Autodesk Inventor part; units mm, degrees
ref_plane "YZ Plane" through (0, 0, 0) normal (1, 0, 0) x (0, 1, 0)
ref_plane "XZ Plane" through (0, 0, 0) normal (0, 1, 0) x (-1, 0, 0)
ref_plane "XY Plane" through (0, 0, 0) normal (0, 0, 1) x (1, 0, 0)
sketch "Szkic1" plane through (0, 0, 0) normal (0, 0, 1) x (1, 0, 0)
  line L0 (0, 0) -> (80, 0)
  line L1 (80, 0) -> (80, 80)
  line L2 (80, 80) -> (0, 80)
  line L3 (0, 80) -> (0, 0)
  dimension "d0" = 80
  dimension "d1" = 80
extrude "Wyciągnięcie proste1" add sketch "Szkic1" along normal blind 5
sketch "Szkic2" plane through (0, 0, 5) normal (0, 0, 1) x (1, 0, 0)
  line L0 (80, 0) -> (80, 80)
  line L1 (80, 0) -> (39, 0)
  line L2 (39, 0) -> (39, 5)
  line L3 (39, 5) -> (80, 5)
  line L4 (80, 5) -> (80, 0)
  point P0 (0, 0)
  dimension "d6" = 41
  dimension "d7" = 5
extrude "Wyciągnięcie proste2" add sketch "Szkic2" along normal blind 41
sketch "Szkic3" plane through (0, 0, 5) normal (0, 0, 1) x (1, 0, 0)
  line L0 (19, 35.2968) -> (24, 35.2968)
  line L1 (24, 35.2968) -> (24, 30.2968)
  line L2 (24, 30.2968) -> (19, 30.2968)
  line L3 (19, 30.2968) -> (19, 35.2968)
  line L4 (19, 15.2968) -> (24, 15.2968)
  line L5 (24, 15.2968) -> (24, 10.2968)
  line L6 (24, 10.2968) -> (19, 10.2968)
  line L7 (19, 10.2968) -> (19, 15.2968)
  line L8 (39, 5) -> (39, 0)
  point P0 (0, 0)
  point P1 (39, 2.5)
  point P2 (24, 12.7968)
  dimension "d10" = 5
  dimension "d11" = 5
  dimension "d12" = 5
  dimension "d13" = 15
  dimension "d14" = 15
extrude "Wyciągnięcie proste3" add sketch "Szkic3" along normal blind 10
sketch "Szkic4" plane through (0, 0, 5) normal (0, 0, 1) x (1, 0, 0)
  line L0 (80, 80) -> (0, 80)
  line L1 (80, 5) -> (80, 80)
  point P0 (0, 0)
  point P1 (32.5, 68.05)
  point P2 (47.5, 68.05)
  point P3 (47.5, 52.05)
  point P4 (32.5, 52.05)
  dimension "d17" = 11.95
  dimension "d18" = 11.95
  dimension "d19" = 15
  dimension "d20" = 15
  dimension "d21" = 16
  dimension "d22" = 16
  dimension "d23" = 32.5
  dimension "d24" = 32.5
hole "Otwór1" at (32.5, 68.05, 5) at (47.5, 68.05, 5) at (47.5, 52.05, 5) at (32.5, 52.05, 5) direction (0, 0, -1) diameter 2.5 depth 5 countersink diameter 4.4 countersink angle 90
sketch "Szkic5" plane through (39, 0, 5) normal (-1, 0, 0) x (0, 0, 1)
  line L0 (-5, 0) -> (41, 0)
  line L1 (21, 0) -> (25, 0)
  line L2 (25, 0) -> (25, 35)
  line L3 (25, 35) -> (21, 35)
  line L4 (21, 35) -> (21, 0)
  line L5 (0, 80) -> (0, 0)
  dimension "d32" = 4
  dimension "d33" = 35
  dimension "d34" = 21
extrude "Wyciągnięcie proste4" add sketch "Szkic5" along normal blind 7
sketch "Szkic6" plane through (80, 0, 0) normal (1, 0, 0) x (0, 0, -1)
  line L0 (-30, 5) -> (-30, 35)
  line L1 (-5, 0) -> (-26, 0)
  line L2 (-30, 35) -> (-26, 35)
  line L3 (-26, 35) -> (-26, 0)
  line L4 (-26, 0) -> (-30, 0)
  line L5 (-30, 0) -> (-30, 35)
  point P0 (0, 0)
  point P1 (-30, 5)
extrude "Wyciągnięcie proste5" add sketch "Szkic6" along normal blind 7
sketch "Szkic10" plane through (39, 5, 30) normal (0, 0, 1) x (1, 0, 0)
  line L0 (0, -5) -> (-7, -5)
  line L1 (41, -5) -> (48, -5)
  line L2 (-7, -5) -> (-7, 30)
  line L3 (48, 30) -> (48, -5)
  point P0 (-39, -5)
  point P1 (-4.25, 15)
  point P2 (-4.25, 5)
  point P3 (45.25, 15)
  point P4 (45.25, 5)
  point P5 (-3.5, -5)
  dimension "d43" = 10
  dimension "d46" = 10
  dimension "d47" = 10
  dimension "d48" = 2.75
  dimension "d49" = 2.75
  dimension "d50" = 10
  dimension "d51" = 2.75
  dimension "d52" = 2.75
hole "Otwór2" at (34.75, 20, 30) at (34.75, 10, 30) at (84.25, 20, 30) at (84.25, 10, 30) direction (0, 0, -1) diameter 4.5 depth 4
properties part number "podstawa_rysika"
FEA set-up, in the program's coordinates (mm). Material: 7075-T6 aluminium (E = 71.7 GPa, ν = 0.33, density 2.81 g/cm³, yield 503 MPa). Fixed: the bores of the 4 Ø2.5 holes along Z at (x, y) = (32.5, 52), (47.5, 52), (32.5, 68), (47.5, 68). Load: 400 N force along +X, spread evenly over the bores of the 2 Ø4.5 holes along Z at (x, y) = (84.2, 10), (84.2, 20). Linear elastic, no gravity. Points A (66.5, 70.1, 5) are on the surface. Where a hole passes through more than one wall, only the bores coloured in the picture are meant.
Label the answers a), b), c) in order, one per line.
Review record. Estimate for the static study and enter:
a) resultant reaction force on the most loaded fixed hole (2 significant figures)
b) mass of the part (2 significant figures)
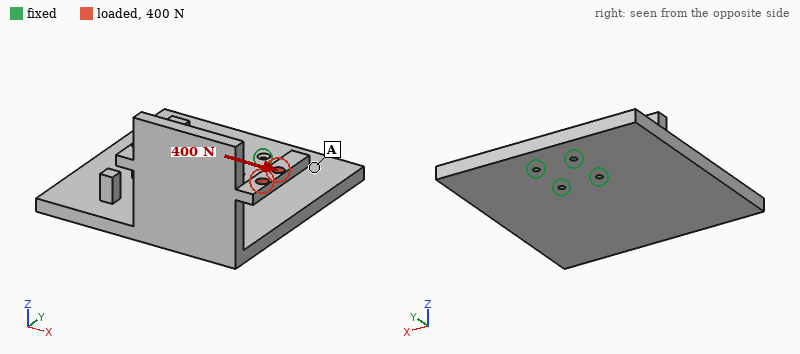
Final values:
a) 720 N
b) 120 g
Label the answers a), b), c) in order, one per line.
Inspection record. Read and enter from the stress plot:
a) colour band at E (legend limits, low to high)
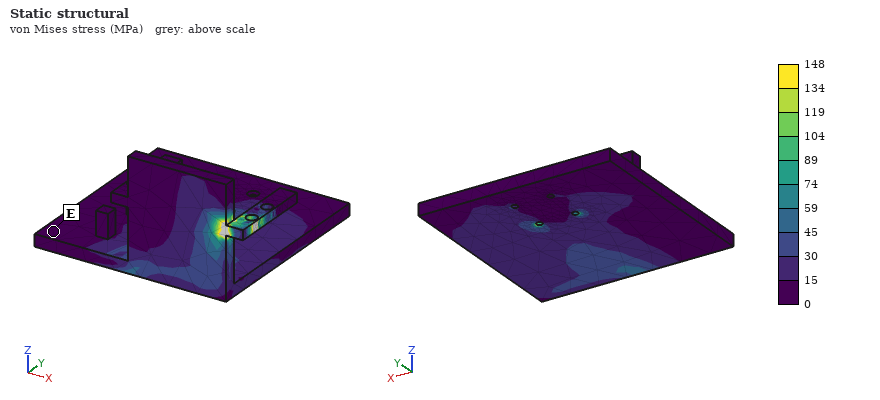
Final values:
a) 0 to 15 MPa
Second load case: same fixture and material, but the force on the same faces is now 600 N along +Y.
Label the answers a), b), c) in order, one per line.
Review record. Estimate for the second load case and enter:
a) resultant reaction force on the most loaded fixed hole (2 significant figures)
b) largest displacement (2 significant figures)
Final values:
a) 810 N
b) 1.2 mm
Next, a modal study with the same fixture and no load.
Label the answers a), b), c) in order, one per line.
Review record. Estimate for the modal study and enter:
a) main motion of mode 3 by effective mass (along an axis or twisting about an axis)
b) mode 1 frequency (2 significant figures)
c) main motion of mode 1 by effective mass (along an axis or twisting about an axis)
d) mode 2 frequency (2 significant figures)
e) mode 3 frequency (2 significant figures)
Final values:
a) along Z
b) 650 Hz
c) along Z
d) 1000 Hz
e) 1400 Hz
